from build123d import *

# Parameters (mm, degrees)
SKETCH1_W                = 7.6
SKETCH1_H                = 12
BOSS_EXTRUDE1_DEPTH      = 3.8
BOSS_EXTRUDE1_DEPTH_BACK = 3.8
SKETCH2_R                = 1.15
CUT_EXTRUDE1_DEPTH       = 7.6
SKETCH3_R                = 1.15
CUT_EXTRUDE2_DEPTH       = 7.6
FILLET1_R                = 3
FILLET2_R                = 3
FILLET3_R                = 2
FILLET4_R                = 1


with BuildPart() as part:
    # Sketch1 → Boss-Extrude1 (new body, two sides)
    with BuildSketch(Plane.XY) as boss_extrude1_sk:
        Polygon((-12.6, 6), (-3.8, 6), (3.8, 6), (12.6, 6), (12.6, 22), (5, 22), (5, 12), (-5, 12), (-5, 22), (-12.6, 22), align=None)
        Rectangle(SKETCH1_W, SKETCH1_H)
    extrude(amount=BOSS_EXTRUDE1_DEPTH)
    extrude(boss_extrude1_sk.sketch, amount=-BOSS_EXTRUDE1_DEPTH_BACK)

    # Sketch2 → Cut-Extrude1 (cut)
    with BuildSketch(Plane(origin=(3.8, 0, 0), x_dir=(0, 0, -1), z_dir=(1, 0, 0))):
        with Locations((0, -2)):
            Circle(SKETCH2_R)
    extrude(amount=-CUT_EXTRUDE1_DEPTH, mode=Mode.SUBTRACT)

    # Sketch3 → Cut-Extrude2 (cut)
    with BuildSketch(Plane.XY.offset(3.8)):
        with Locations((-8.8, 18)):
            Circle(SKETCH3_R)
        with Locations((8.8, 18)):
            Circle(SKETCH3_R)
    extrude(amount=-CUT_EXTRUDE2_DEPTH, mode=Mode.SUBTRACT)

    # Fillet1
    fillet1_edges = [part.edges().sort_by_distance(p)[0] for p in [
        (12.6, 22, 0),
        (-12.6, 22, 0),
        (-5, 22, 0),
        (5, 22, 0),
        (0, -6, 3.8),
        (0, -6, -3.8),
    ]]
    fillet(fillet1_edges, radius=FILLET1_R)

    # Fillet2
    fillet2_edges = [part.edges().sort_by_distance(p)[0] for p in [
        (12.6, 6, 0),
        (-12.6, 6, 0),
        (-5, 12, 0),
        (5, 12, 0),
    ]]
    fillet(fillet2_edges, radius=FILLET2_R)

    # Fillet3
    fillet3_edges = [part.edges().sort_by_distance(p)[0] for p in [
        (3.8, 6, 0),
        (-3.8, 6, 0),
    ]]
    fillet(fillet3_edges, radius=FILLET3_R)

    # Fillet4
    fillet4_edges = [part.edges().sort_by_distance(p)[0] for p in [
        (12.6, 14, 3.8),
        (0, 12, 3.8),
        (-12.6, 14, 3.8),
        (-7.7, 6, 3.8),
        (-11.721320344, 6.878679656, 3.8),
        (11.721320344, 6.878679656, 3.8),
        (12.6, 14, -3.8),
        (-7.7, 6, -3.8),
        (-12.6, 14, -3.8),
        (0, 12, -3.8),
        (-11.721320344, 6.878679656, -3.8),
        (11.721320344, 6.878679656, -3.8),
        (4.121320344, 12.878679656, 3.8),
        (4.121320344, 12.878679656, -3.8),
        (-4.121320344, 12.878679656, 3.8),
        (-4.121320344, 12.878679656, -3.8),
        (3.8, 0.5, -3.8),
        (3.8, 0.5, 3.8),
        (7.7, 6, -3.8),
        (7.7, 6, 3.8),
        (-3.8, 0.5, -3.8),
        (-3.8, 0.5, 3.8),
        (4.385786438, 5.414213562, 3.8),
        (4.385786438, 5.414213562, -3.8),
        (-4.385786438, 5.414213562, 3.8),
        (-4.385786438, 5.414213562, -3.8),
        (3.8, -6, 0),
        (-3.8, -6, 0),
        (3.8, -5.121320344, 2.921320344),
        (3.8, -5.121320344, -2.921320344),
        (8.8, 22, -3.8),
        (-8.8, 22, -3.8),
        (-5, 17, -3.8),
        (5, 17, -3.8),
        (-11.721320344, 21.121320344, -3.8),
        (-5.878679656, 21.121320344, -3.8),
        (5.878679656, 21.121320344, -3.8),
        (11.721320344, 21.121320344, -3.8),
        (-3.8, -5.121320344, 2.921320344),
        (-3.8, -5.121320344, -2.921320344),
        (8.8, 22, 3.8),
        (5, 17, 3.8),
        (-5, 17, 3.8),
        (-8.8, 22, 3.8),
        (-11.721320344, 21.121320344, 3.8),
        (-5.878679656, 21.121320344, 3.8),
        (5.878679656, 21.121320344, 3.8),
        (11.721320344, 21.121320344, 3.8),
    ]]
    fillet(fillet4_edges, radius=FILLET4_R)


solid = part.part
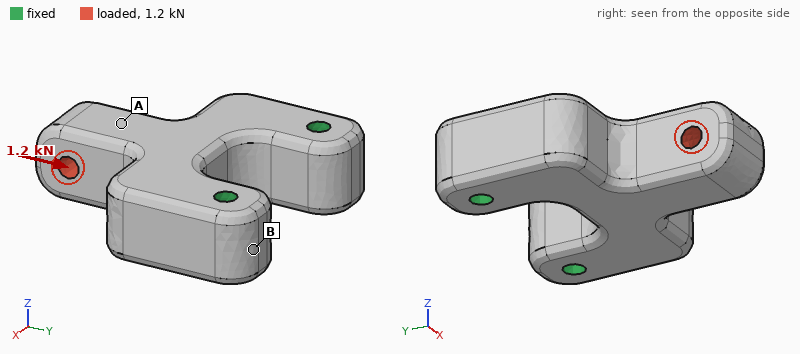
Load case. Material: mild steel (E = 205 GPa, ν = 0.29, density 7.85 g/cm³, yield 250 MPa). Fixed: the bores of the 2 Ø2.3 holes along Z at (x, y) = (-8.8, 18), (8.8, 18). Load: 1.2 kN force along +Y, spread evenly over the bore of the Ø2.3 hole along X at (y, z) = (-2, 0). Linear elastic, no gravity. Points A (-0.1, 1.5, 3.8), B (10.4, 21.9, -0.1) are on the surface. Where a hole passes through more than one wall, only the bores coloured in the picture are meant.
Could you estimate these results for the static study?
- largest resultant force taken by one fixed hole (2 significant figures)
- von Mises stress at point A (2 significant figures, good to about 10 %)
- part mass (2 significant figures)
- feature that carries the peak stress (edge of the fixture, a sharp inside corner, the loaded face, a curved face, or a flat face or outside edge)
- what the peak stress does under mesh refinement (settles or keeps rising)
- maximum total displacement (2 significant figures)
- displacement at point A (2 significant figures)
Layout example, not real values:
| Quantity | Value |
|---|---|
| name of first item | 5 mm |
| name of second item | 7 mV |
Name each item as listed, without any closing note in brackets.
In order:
| Quantity | Value |
|---|---|
| largest resultant force taken by one fixed hole | 660 N |
| von Mises stress at point A | 18 MPa |
| part mass | 22 g |
| feature that carries the peak stress | a sharp inside corner |
| what the peak stress does under mesh refinement | keeps rising |
| maximum total displacement | 2.5 µm |
| displacement at point A | 1.7 µm |
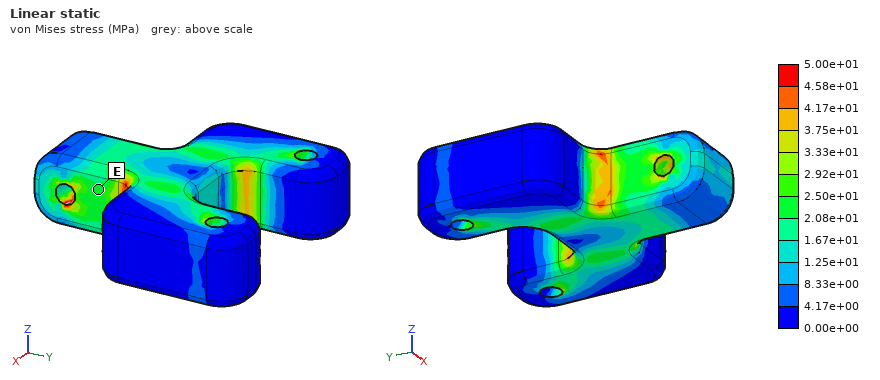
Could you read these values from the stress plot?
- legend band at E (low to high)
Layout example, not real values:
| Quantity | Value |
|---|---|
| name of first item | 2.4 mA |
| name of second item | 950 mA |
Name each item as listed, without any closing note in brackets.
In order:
| Quantity | Value |
|---|---|
| legend band at E | 2.08e+01 to 2.50e+01 MPa |
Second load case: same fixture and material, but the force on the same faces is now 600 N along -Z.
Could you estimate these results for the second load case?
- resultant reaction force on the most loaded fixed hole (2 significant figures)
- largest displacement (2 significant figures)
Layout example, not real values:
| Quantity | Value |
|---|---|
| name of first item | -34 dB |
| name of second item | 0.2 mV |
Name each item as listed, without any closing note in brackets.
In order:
| Quantity | Value |
|---|---|
| resultant reaction force on the most loaded fixed hole | 300 N |
| largest displacement | 29 µm |
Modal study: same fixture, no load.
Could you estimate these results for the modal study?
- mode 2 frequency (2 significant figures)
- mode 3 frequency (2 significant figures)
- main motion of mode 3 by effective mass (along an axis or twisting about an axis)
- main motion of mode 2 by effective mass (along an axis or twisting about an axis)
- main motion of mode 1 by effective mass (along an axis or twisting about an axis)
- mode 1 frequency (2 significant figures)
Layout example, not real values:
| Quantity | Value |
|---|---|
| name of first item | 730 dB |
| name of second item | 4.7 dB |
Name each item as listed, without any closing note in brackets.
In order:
| Quantity | Value |
|---|---|
| mode 2 frequency | 26 kHz |
| mode 3 frequency | 38 kHz |
| main motion of mode 3 by effective mass | along X |
| main motion of mode 2 by effective mass | along X |
| main motion of mode 1 by effective mass | along Z |
| mode 1 frequency | 12 kHz |
